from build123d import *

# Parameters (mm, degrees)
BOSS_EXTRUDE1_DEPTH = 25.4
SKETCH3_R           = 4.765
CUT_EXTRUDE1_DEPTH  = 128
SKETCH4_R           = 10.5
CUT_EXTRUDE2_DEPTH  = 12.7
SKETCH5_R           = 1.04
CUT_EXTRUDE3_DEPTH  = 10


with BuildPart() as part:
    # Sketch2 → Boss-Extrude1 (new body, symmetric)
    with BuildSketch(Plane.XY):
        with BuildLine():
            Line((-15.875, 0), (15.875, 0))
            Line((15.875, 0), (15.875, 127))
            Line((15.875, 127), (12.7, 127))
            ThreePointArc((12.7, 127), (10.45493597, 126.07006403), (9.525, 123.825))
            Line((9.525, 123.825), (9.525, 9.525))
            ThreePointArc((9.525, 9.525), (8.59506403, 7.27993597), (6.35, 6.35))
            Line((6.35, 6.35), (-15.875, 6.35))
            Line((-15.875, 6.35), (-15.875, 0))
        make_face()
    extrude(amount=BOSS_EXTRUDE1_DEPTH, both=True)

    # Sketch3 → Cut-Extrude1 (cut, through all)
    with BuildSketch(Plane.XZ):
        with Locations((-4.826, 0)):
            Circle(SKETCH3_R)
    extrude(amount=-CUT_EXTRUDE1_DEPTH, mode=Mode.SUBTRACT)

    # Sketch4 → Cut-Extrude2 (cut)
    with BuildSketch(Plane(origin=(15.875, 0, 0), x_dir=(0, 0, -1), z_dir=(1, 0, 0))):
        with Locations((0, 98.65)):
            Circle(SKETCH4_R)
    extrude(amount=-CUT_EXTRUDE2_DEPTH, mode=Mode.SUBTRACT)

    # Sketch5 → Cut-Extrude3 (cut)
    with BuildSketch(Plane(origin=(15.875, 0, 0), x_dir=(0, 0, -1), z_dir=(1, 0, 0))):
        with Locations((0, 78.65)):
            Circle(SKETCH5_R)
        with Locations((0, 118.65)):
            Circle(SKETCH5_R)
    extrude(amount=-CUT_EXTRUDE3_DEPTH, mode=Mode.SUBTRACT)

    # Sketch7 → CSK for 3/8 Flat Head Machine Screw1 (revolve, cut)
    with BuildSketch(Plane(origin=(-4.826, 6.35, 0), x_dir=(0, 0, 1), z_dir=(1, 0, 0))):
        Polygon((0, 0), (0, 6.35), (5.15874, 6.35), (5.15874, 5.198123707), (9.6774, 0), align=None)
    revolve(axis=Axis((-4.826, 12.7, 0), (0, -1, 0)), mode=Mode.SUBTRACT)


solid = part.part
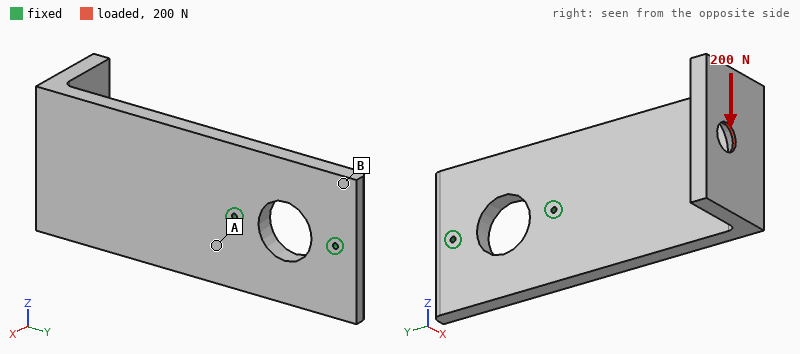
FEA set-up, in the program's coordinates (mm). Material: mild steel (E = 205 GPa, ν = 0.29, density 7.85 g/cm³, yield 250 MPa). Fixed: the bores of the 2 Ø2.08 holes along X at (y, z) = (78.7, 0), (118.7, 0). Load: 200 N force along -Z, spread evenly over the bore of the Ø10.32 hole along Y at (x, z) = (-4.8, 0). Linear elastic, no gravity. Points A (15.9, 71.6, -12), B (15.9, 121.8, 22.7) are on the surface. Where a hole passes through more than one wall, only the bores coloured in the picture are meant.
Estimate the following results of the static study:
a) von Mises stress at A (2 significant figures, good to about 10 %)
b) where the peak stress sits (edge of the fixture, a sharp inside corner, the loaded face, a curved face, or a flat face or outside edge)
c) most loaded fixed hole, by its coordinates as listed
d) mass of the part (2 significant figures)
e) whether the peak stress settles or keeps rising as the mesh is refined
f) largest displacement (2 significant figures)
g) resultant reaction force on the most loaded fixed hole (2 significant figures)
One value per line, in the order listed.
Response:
6.3 MPa
edge of the fixture
(78.7, 0)
360 g
keeps rising
41 µm
570 N
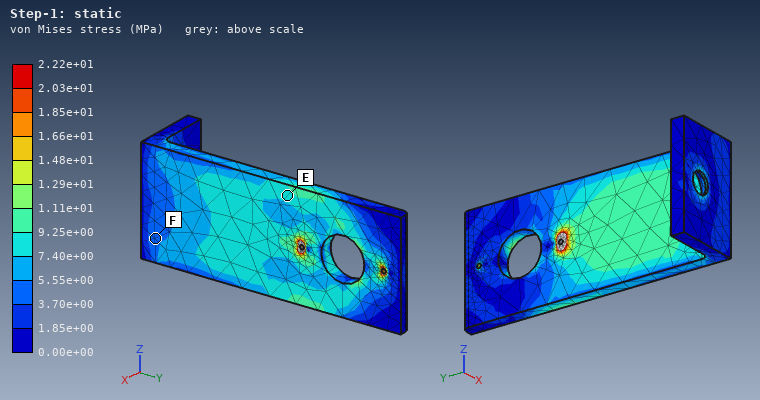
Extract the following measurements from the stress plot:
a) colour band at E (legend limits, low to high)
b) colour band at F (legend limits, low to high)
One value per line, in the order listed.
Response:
7.40e+00 to 9.25e+00 MPa
3.70e+00 to 5.55e+00 MPa
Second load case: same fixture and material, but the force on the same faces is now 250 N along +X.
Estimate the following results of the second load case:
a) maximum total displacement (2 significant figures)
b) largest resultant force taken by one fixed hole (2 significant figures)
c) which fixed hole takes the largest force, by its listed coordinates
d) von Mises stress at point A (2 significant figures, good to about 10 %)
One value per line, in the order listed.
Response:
0.25 mm
530 N
(78.7, 0)
47 MPa
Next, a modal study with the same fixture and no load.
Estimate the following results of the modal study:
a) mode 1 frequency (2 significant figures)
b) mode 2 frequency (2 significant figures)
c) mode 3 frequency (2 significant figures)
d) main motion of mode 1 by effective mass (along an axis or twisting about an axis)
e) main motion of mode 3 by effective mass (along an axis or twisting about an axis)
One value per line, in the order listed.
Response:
510 Hz
1300 Hz
2400 Hz
along X
along Z
